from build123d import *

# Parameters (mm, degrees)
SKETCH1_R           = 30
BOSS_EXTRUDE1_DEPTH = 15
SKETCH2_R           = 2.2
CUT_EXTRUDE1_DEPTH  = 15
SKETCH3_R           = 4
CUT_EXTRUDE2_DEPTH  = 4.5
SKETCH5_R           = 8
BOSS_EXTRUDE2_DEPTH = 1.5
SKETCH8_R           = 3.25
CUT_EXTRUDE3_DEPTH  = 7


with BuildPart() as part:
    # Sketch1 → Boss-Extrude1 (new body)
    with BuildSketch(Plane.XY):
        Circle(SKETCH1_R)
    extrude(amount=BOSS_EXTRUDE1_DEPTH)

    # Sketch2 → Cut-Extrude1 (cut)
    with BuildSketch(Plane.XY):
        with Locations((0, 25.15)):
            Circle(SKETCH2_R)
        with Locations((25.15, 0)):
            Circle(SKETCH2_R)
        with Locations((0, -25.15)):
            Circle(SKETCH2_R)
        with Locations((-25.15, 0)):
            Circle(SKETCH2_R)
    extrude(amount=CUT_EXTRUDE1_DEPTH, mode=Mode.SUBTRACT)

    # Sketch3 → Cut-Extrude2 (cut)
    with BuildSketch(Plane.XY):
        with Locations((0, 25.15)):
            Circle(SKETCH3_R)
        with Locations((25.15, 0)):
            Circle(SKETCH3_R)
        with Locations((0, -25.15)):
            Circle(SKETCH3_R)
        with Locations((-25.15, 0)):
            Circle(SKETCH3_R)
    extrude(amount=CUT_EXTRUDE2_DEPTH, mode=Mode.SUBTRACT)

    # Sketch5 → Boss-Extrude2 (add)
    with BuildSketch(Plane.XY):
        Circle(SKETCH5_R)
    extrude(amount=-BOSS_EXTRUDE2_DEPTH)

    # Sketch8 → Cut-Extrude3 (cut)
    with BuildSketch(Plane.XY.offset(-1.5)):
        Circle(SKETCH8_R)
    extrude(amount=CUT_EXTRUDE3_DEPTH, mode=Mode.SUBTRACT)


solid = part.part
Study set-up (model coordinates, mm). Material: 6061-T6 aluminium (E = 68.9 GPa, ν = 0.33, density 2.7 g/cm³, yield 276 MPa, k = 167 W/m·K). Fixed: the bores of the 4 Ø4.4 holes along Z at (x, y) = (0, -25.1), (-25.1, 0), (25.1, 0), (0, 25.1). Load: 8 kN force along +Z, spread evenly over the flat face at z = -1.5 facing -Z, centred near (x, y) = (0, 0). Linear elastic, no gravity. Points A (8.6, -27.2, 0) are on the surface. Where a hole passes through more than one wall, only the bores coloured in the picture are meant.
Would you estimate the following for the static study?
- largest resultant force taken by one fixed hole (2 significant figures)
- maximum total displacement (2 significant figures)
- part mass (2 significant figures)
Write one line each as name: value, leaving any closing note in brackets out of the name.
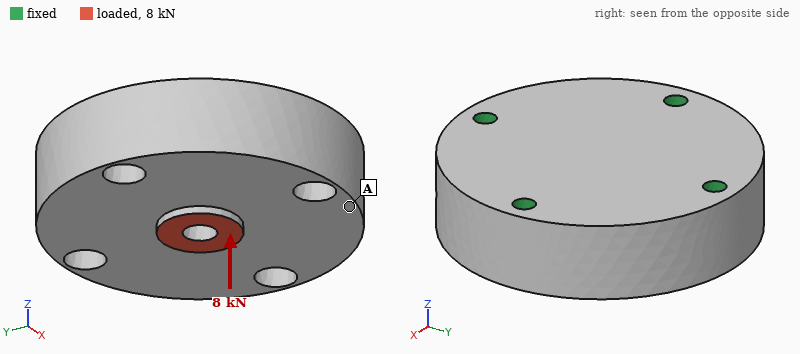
largest resultant force taken by one fixed hole: 2.2 kN
maximum total displacement: 16 µm
part mass: 110 g
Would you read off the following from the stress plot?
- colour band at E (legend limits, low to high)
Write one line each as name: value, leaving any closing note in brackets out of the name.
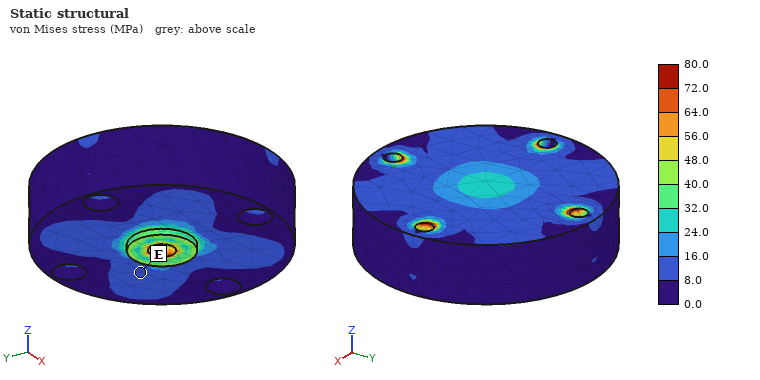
colour band at E: 8.0 to 16.0 MPa
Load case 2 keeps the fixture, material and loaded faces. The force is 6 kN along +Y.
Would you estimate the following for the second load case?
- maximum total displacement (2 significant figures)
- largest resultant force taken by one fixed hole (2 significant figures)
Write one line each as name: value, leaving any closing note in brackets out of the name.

maximum total displacement: 13 µm
largest resultant force taken by one fixed hole: 2.4 kN
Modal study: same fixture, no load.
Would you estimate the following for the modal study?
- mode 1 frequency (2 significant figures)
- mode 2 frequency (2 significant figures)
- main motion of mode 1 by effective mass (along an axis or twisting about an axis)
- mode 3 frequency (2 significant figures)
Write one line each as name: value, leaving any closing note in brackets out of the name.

mode 1 frequency: 23 kHz
mode 2 frequency: 25 kHz
main motion of mode 1 by effective mass: along Z
mode 3 frequency: 26 kHz
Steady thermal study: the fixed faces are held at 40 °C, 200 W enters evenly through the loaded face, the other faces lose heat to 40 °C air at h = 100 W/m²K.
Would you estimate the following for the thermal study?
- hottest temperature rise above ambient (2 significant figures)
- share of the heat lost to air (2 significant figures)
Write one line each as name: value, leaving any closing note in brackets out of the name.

hottest temperature rise above ambient: 54 K
share of the heat lost to air: 3.9 %
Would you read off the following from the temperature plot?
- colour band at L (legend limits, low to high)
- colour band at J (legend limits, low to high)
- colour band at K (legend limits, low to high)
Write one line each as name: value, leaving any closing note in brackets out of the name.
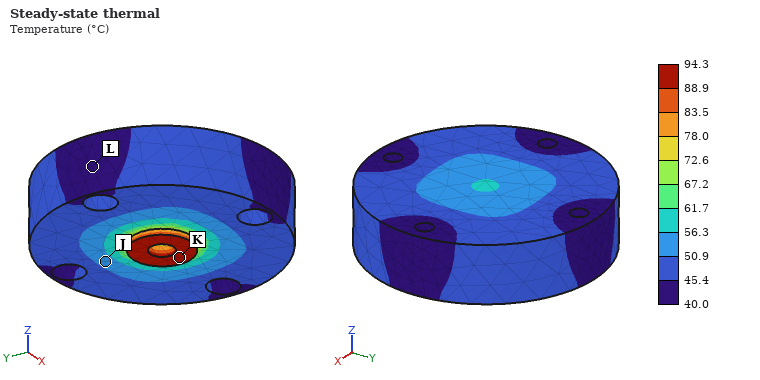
colour band at L: 40.0 to 45.4 °C
colour band at J: 50.9 to 56.3 °C
colour band at K: 88.9 to 94.3 °C
